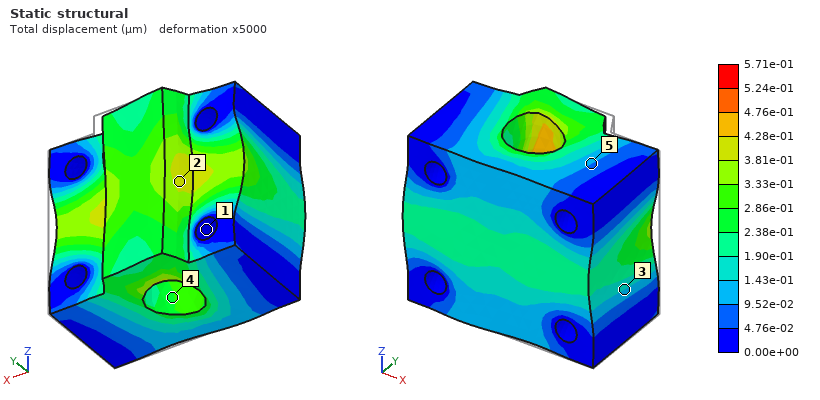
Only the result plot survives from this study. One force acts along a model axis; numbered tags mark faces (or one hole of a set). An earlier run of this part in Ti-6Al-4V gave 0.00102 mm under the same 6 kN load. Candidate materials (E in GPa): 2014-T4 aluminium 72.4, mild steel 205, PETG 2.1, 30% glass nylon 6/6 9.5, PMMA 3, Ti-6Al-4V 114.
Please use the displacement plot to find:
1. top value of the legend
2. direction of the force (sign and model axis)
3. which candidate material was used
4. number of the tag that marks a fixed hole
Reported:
5.71e-01 µm
-X
mild steel
1
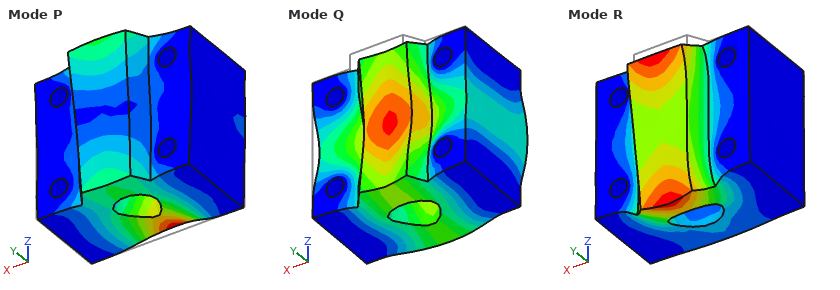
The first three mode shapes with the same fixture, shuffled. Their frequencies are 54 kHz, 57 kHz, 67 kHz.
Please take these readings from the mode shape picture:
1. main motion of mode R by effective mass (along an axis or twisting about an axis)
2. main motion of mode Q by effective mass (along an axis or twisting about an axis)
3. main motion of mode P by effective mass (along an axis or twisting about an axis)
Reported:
along Z
along Y
along Z
